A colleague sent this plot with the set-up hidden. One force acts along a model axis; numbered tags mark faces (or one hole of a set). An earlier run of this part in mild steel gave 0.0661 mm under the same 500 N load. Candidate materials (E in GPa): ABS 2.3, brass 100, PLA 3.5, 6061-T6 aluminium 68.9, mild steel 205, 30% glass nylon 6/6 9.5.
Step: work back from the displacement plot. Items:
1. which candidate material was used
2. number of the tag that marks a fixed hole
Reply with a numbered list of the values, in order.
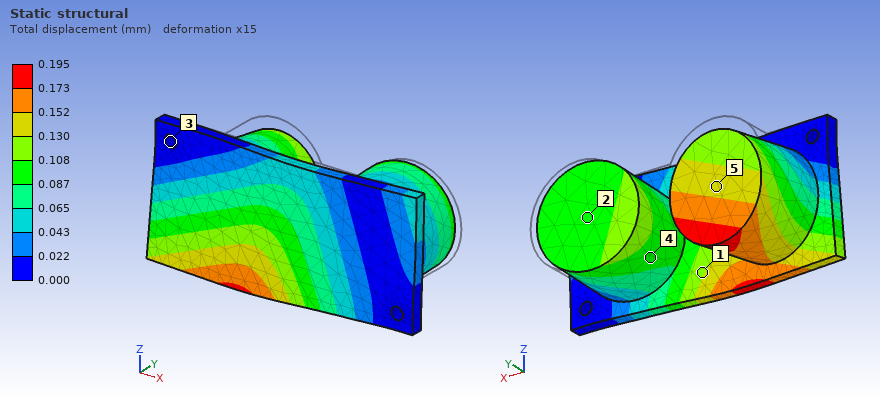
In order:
1. 6061-T6 aluminium
2. 3
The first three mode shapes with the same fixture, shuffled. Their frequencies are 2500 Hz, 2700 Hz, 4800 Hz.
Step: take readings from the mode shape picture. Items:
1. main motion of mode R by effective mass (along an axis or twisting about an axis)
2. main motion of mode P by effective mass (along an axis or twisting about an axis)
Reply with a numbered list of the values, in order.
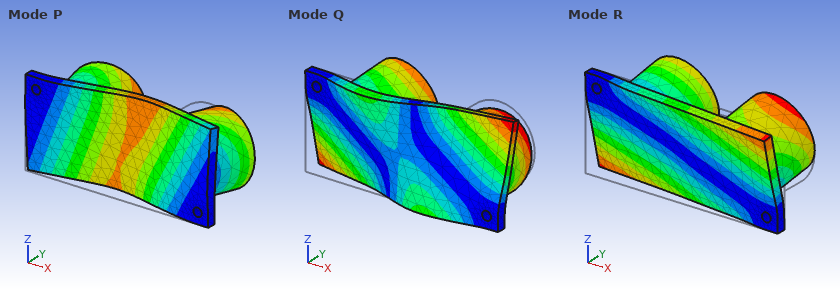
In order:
1. along Z
2. along Y
